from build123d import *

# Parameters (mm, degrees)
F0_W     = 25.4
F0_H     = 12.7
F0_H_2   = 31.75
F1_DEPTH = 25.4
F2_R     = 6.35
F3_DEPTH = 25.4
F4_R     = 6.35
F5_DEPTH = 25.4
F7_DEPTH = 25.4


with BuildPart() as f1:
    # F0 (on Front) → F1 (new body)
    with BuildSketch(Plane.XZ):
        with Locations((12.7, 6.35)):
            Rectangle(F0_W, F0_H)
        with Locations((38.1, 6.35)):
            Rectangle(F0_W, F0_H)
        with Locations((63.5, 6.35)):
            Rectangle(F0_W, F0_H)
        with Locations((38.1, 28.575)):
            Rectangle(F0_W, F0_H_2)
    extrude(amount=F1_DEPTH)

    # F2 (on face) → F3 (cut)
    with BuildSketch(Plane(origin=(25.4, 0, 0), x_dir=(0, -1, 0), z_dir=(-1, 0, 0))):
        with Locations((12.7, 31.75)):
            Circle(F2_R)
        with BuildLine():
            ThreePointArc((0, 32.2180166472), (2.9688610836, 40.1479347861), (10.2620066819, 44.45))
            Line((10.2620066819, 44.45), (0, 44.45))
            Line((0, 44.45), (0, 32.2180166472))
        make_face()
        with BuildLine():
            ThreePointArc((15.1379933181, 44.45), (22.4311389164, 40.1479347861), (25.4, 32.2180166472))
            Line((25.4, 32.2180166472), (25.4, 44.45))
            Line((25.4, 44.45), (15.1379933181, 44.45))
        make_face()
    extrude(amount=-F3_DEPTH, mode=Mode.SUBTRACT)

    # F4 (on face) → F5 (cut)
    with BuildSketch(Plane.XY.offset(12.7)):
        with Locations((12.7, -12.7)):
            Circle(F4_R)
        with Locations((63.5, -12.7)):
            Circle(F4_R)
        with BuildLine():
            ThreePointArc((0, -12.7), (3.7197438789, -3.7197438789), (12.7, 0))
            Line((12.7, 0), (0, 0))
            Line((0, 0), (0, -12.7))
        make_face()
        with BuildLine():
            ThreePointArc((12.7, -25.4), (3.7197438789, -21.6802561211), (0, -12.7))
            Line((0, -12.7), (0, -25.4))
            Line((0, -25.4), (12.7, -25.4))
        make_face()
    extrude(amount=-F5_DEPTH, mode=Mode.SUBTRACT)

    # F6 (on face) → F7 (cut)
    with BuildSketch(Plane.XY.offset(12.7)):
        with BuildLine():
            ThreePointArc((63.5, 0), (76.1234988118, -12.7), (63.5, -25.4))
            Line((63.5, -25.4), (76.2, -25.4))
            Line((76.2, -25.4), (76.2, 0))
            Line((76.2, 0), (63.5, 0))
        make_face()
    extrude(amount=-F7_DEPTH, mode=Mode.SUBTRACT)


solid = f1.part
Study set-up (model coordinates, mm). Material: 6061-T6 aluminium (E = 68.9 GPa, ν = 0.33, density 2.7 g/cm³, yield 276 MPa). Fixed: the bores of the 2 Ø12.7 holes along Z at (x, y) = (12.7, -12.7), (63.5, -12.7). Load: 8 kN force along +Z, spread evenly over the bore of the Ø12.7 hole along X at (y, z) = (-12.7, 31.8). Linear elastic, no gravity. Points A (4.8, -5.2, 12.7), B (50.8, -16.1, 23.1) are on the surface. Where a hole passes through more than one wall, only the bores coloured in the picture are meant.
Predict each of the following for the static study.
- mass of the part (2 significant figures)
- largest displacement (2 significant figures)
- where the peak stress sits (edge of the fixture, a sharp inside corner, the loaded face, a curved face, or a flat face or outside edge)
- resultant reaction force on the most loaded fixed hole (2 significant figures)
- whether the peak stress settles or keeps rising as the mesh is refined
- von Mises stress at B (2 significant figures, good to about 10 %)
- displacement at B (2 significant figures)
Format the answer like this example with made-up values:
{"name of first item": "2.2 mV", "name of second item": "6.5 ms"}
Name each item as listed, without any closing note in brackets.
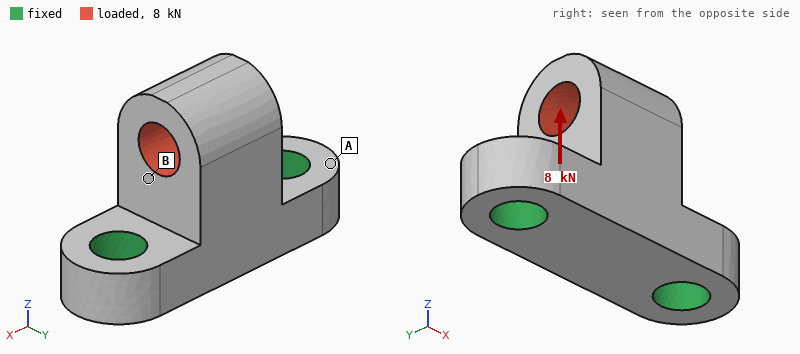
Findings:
{"mass of the part": "95 g", "largest displacement": "18 µm", "where the peak stress sits": "edge of the fixture", "resultant reaction force on the most loaded fixed hole": "4.2 kN", "whether the peak stress settles or keeps rising as the mesh is refined": "keeps rising", "von Mises stress at B": "15 MPa", "displacement at B": "11 µm"}
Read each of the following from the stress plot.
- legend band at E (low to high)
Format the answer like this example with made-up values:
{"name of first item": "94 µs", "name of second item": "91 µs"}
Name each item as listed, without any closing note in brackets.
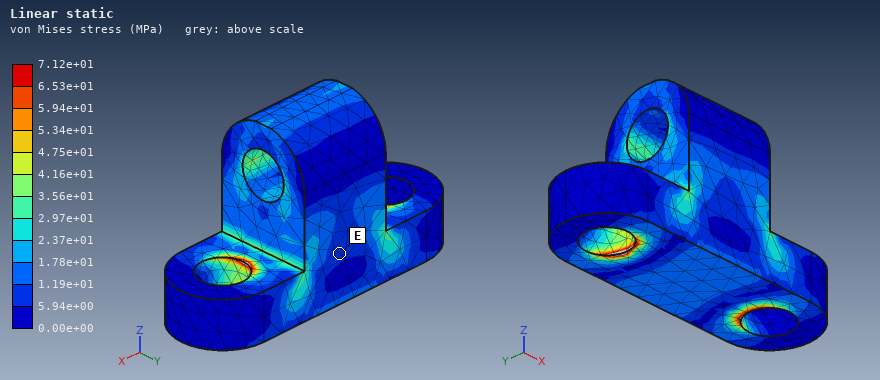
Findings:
{"legend band at E": "5.94e+00 to 1.19e+01 MPa"}
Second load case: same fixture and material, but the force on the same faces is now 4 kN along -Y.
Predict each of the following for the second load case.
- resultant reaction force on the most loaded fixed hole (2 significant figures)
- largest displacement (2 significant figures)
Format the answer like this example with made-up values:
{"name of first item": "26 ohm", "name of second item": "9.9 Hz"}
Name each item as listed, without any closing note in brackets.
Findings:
{"resultant reaction force on the most loaded fixed hole": "2.0 kN", "largest displacement": "88 µm"}
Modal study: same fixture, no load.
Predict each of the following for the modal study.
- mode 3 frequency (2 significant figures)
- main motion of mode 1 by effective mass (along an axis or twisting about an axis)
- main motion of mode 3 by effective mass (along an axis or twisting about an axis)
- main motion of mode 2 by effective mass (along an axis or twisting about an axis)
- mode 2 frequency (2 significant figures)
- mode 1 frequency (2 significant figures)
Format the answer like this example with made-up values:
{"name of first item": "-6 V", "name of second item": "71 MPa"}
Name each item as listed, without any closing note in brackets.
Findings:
{"mode 3 frequency": "17 kHz", "main motion of mode 1 by effective mass": "along Y", "main motion of mode 3 by effective mass": "along Z", "main motion of mode 2 by effective mass": "along X", "mode 2 frequency": "12 kHz", "mode 1 frequency": "6900 Hz"}
